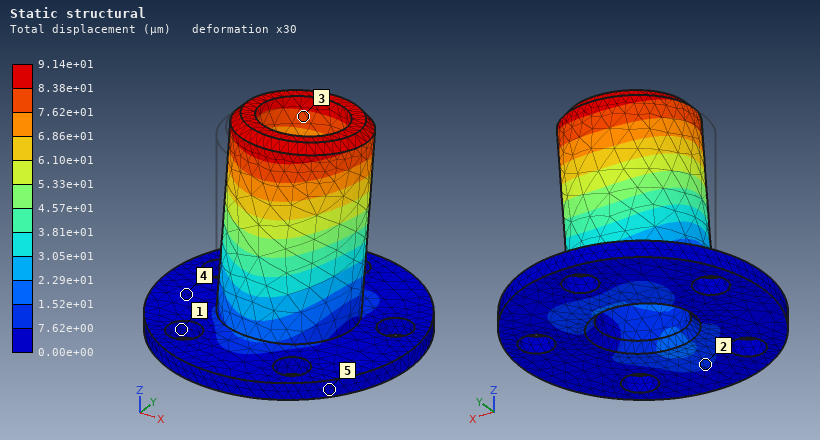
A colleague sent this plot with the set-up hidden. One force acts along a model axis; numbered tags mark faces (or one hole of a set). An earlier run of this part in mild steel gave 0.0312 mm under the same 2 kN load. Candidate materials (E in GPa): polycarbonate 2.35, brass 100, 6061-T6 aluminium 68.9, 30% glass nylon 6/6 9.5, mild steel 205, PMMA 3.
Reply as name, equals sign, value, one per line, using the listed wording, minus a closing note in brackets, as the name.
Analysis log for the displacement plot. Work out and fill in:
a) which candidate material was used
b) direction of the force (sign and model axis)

which candidate material was used = 6061-T6 aluminium
direction of the force = +Y
